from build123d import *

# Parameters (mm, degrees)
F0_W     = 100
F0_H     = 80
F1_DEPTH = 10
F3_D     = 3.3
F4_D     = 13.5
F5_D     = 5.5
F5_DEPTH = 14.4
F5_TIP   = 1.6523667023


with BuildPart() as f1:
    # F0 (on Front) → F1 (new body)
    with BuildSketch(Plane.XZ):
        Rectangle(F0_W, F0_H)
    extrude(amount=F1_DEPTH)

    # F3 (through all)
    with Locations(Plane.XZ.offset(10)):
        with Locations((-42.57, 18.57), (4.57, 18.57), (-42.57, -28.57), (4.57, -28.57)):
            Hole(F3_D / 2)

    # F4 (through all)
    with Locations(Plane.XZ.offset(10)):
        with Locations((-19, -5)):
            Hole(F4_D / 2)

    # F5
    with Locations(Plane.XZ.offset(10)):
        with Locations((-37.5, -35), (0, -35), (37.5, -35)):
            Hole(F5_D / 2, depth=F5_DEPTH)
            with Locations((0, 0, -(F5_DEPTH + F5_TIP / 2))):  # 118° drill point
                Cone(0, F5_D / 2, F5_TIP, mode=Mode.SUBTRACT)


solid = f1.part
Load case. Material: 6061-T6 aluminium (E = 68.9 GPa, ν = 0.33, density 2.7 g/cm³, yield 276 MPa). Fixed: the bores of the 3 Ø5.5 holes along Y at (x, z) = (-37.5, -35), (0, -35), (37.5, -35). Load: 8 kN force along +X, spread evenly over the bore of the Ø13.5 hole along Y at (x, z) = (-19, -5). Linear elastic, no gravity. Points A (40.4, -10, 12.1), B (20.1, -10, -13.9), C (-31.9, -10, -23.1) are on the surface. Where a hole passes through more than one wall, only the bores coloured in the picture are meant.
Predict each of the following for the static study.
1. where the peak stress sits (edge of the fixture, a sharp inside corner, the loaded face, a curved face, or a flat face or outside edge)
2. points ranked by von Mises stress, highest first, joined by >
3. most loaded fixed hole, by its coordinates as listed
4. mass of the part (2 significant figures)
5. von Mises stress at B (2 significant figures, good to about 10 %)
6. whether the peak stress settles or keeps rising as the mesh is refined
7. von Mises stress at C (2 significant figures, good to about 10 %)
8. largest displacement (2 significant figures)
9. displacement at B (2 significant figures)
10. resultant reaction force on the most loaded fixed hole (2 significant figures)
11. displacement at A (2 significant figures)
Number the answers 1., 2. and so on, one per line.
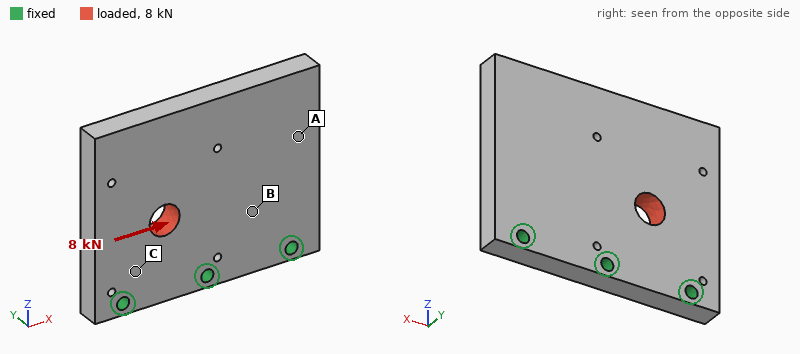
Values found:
1. edge of the fixture
2. C > B > A
3. (-37.5, -35)
4. 210 g
5. 13 MPa
6. keeps rising
7. 24 MPa
8. 22 µm
9. 8.2 µm
10. 4.1 kN
11. 16 µm
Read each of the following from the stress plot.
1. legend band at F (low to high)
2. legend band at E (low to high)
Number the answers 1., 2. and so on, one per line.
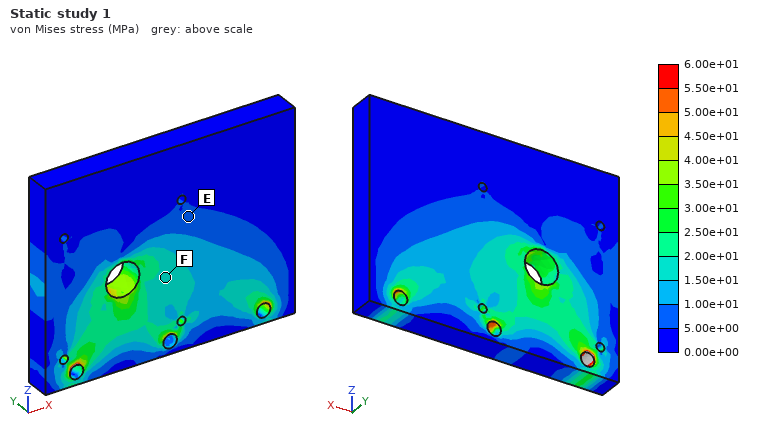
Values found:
1. 1.50e+01 to 2.00e+01 MPa
2. 5.00e+00 to 1.00e+01 MPa
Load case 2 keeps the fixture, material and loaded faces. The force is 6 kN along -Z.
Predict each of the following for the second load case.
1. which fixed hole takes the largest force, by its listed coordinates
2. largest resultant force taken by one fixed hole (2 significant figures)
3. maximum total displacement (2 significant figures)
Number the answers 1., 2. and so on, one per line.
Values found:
1. (-37.5, -35)
2. 3.4 kN
3. 9.3 µm
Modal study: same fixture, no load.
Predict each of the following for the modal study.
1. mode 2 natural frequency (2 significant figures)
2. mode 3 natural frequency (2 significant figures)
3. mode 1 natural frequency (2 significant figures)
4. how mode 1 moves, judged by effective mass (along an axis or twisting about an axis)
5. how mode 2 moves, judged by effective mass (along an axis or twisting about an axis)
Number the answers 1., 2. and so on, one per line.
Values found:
1. 2600 Hz
2. 6500 Hz
3. 1300 Hz
4. along Y
5. twisting about Z
